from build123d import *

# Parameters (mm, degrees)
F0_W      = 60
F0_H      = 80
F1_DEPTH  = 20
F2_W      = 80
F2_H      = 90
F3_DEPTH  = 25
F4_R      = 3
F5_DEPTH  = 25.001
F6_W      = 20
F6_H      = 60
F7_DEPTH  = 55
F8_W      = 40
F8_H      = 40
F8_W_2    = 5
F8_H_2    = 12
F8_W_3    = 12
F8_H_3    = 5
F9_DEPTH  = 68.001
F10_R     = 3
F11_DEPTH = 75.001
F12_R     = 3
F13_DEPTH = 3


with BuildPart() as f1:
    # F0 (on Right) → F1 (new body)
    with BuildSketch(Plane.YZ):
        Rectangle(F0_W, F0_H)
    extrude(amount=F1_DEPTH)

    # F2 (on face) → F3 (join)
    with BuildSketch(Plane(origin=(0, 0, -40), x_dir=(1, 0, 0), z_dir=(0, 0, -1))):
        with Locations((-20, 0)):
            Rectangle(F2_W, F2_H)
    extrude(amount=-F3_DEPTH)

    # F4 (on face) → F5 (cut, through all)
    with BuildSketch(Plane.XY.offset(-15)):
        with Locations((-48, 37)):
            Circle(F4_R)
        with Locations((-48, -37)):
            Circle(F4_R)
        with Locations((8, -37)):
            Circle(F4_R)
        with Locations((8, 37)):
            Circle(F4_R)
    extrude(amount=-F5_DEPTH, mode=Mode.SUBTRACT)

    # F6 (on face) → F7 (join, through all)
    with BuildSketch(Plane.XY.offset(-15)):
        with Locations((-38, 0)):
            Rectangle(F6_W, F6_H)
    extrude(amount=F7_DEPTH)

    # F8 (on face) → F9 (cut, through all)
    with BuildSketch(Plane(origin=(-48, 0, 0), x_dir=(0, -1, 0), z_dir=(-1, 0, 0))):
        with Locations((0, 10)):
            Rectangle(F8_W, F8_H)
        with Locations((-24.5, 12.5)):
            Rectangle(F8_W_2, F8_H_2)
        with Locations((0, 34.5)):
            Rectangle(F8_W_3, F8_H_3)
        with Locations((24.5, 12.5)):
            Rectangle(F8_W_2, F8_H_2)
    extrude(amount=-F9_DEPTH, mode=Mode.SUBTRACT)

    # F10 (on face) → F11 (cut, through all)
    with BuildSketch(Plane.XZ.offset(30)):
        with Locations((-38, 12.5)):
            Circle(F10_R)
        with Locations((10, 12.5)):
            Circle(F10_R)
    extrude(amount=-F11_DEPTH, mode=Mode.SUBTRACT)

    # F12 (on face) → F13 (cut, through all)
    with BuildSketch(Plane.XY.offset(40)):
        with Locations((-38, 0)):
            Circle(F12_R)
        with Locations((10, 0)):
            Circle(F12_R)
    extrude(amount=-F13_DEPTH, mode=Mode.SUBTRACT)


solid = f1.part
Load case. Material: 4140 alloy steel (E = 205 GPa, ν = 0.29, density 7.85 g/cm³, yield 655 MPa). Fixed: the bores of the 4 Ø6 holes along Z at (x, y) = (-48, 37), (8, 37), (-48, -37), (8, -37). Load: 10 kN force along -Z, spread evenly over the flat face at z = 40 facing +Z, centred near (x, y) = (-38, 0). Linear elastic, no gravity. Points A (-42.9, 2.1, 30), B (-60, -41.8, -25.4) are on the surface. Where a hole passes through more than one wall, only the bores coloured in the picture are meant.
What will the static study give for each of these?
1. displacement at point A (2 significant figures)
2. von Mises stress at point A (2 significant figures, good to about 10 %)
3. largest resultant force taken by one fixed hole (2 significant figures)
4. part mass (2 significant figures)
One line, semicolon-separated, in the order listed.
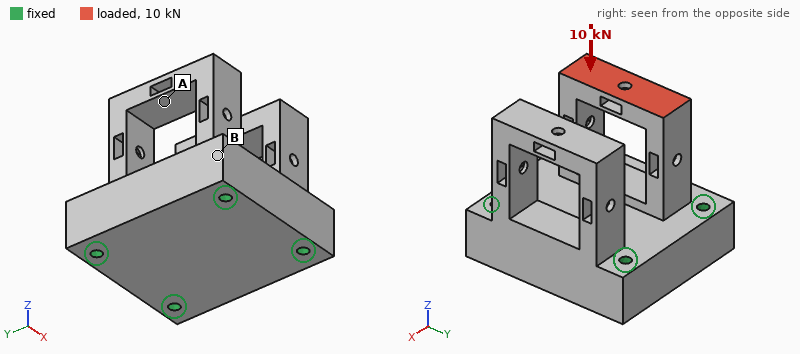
33 µm; 93 MPa; 4.1 kN; 1.9 kg
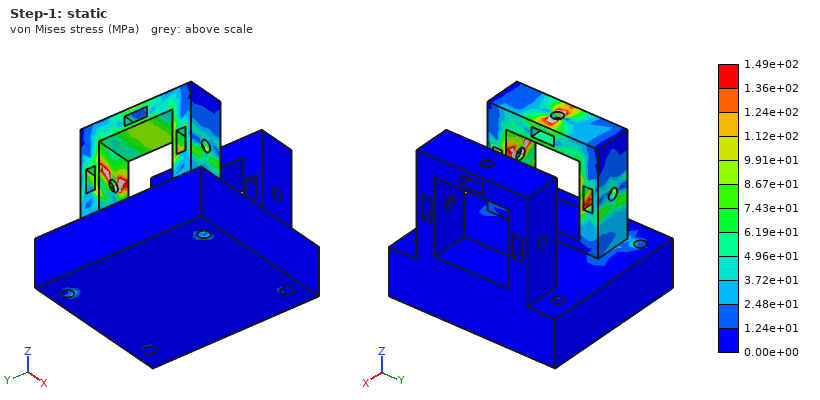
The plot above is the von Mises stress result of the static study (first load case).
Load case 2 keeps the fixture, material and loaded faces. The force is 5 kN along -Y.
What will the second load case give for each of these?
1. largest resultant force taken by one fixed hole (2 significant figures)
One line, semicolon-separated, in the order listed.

4.3 kN
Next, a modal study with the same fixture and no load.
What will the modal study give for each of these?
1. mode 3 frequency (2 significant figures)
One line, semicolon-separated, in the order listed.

2900 Hz
